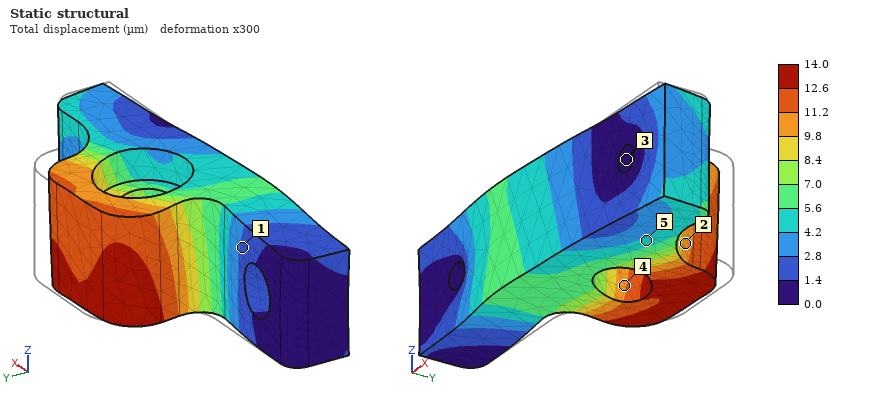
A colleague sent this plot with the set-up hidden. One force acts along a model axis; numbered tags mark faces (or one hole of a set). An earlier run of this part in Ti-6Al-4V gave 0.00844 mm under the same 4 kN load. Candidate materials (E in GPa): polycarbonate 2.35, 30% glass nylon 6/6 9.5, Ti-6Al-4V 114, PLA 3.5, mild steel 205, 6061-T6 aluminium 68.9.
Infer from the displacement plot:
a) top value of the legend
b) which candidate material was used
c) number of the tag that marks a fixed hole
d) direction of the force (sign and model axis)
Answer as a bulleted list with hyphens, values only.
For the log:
- 14.0 µm
- 6061-T6 aluminium
- 3
- -X
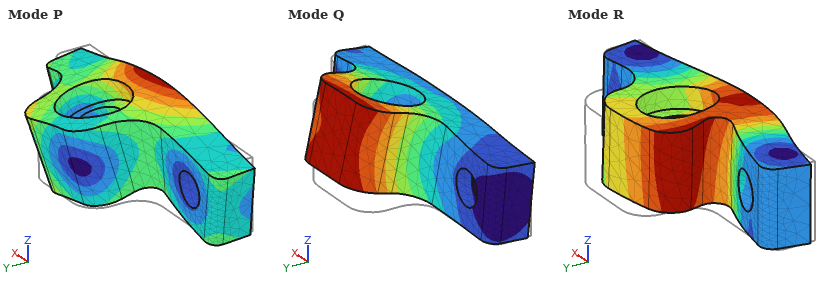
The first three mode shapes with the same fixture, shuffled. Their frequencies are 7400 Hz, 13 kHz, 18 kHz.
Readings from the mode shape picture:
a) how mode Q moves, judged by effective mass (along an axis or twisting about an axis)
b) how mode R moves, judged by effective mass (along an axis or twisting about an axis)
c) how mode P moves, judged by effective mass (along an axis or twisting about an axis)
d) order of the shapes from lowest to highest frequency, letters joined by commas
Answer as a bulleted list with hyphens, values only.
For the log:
- along Z
- along Y
- along Z
- Q, R, P
